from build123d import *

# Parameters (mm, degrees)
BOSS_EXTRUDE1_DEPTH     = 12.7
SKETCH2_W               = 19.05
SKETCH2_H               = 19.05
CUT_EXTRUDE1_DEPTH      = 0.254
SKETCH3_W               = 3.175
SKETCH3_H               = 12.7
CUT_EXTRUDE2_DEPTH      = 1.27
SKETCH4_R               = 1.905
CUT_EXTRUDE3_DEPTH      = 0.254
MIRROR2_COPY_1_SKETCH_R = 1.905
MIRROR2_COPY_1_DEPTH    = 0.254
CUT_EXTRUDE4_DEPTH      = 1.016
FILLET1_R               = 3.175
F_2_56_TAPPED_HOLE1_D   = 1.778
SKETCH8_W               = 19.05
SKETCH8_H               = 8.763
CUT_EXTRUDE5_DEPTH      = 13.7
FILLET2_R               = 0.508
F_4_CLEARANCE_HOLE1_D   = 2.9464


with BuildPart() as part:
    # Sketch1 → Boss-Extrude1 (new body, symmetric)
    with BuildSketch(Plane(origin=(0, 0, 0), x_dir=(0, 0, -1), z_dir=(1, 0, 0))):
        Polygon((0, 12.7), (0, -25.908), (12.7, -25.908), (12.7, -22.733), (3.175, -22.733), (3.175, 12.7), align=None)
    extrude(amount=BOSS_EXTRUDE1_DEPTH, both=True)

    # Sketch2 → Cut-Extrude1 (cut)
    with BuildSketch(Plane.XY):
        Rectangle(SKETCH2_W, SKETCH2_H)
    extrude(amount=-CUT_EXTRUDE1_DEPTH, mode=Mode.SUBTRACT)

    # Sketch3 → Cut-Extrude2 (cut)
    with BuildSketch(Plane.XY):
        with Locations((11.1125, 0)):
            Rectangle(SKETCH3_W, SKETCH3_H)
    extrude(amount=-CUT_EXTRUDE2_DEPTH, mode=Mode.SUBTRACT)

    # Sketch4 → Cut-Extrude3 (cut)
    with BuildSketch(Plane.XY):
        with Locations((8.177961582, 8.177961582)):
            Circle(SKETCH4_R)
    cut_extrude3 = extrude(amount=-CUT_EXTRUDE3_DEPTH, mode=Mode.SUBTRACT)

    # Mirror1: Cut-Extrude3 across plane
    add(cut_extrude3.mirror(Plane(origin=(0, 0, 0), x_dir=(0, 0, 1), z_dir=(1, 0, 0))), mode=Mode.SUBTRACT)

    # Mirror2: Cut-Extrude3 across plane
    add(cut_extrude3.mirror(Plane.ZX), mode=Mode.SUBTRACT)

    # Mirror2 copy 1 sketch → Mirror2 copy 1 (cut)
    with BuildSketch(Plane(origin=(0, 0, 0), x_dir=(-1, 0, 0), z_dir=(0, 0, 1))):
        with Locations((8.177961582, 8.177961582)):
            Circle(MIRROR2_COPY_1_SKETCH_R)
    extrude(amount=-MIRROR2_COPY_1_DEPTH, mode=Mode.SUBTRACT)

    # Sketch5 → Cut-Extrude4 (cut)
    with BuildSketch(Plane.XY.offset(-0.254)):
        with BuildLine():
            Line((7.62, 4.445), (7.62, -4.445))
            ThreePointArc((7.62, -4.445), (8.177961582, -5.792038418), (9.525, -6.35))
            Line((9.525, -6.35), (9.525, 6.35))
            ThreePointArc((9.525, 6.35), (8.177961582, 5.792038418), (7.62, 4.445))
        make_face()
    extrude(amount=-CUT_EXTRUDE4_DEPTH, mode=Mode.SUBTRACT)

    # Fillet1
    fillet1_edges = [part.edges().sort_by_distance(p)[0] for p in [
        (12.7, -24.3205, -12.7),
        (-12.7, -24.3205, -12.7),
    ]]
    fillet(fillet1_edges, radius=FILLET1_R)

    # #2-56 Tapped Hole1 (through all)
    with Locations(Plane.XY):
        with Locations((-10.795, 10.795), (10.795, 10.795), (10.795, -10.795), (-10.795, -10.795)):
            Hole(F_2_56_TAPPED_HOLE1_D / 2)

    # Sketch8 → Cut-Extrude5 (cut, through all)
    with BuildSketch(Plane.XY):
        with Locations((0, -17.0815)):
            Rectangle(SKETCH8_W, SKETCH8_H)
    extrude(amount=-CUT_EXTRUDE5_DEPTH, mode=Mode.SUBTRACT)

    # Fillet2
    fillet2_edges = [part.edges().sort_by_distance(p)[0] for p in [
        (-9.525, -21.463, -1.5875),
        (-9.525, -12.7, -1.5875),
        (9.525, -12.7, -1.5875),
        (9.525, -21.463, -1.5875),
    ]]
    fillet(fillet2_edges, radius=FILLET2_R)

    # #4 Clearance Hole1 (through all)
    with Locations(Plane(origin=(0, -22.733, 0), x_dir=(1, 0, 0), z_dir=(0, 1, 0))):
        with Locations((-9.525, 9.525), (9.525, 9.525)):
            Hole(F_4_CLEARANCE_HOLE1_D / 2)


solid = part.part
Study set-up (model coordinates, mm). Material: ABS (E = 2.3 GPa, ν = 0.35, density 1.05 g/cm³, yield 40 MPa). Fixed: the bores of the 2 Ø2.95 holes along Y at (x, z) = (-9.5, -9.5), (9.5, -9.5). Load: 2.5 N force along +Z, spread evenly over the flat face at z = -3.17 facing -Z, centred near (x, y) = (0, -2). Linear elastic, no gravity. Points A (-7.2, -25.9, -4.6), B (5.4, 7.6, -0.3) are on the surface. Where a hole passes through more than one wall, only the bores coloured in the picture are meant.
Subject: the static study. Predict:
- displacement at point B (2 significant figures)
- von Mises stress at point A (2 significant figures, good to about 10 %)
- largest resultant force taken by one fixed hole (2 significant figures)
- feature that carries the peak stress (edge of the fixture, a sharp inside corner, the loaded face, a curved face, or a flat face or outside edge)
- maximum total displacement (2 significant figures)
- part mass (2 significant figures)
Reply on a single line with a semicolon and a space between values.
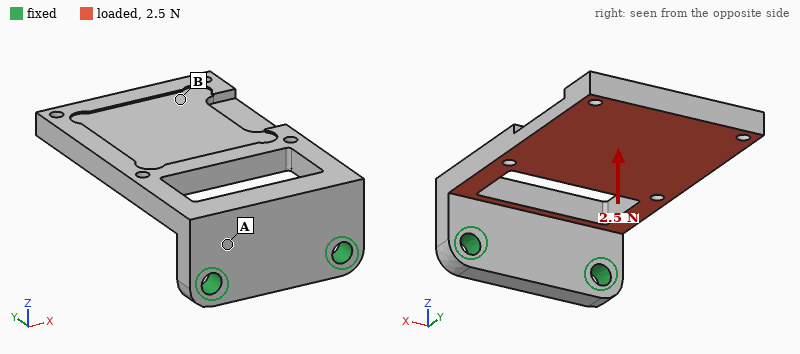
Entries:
0.47 mm; 1.2 MPa; 1.3 N; a curved face; 0.56 mm; 3.3 g
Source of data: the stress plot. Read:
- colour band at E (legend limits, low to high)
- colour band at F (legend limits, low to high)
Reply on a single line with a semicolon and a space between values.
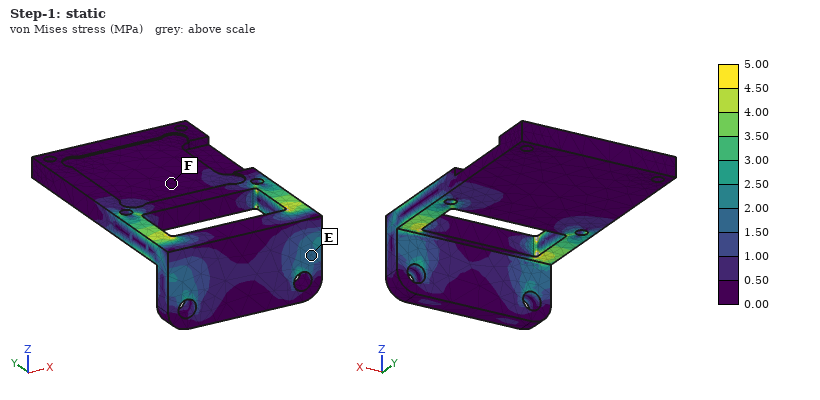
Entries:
1.50 to 2.00 MPa; 0.00 to 0.50 MPa
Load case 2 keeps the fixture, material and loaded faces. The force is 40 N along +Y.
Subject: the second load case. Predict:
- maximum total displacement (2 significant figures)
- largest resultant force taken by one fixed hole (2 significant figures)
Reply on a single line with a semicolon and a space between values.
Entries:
0.49 mm; 20 N
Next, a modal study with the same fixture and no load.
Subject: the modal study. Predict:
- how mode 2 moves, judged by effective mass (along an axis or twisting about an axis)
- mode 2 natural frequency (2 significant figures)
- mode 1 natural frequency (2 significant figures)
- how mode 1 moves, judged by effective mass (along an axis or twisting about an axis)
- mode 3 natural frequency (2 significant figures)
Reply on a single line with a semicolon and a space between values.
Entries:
along X; 1000 Hz; 270 Hz; along Z; 1300 Hz
